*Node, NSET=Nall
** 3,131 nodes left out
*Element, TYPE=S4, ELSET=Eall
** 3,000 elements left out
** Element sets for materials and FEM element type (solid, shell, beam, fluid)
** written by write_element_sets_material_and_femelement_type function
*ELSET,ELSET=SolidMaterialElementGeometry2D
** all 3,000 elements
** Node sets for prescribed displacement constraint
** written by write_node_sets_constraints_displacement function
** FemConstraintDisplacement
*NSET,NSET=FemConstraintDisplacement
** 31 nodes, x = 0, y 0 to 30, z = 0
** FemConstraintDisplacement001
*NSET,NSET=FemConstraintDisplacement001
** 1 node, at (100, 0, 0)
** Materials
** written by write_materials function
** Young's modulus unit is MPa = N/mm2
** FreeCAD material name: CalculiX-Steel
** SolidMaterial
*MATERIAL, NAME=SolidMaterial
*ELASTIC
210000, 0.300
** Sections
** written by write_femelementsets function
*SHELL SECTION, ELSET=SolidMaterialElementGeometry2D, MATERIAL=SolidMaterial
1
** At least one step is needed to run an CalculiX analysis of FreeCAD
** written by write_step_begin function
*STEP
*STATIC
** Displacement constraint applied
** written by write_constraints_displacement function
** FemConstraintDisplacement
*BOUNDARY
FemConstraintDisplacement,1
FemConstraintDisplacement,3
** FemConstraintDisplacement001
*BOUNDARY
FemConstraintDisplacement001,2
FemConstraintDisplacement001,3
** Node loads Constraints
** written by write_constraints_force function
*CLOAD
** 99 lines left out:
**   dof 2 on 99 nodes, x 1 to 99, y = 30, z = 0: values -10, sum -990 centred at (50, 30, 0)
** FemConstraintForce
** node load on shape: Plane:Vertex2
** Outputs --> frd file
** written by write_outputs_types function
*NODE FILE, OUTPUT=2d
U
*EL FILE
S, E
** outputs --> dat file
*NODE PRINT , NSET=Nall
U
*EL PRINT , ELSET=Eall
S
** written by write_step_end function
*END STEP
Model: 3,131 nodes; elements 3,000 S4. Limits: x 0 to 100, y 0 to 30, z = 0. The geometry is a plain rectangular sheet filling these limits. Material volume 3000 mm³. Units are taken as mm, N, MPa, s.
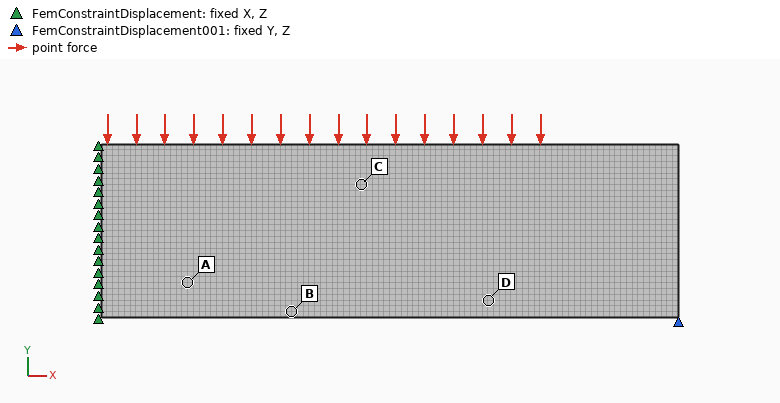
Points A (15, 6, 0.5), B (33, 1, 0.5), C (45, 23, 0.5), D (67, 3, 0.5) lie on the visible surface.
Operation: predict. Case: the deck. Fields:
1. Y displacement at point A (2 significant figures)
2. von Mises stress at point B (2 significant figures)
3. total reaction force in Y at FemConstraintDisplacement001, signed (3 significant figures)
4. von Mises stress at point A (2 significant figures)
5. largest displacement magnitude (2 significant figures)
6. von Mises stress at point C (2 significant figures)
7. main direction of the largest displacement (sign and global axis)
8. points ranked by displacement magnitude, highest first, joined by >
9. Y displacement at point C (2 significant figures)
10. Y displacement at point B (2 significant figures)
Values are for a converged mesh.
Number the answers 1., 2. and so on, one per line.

1. -0.49 mm
2. 280 MPa
3. 990 N
4. 190 MPa
5. 0.51 mm
6. 140 MPa
7. -Y
8. A > B > C > D
9. -0.40 mm
10. -0.45 mm
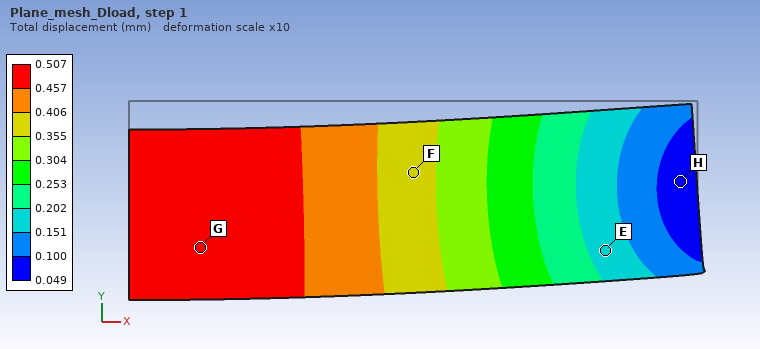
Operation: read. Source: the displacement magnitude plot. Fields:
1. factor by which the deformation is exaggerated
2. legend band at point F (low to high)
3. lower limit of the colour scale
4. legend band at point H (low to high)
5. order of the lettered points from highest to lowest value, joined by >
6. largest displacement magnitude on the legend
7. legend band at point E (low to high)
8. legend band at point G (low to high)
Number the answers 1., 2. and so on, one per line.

1. 10
2. 0.355 to 0.406 mm
3. 0.049 mm
4. 0.049 to 0.100 mm
5. G > F > E > H
6. 0.507 mm
7. 0.151 to 0.202 mm
8. 0.457 to 0.507 mm
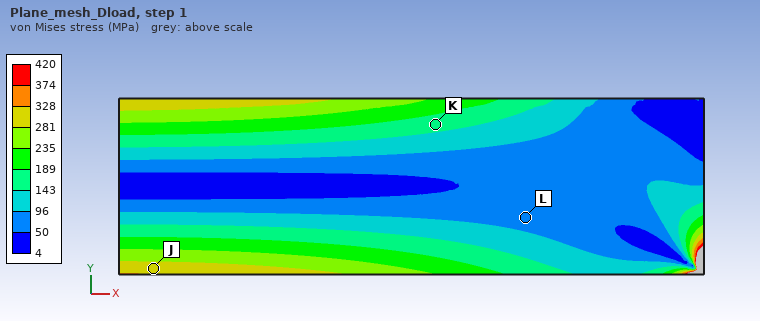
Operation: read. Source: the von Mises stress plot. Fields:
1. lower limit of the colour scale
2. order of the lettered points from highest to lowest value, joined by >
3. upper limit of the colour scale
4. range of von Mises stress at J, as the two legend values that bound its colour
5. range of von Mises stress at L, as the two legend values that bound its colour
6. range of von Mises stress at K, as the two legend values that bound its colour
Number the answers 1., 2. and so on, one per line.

1. 4 MPa
2. J > K > L
3. 420 MPa
4. 281 to 328 MPa
5. 50 to 96 MPa
6. 143 to 189 MPa
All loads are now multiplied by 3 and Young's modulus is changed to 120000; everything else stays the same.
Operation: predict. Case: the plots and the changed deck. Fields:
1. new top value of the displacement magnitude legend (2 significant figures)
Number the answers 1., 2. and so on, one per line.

1. 2.7 mm
